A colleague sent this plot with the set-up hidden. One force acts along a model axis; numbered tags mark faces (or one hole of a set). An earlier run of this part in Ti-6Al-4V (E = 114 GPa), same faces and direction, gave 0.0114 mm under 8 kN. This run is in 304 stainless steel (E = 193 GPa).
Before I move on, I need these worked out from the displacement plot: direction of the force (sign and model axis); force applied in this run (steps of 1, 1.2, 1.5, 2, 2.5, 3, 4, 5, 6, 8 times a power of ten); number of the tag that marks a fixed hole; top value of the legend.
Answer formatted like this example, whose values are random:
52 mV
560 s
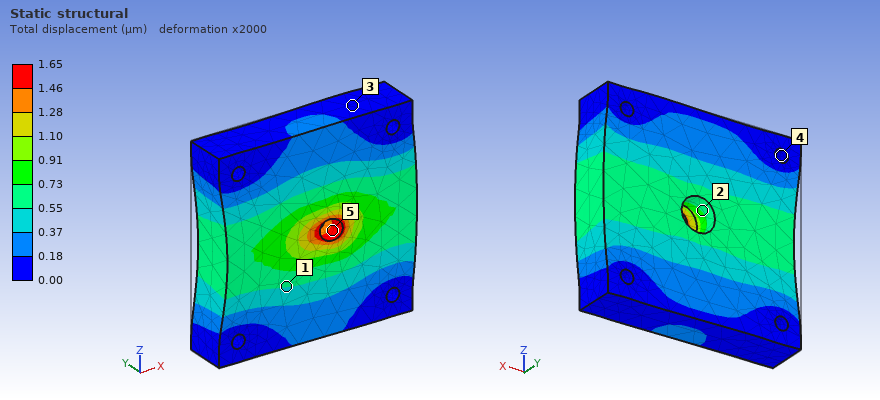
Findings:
+X
2 kN
4
1.65 µm
